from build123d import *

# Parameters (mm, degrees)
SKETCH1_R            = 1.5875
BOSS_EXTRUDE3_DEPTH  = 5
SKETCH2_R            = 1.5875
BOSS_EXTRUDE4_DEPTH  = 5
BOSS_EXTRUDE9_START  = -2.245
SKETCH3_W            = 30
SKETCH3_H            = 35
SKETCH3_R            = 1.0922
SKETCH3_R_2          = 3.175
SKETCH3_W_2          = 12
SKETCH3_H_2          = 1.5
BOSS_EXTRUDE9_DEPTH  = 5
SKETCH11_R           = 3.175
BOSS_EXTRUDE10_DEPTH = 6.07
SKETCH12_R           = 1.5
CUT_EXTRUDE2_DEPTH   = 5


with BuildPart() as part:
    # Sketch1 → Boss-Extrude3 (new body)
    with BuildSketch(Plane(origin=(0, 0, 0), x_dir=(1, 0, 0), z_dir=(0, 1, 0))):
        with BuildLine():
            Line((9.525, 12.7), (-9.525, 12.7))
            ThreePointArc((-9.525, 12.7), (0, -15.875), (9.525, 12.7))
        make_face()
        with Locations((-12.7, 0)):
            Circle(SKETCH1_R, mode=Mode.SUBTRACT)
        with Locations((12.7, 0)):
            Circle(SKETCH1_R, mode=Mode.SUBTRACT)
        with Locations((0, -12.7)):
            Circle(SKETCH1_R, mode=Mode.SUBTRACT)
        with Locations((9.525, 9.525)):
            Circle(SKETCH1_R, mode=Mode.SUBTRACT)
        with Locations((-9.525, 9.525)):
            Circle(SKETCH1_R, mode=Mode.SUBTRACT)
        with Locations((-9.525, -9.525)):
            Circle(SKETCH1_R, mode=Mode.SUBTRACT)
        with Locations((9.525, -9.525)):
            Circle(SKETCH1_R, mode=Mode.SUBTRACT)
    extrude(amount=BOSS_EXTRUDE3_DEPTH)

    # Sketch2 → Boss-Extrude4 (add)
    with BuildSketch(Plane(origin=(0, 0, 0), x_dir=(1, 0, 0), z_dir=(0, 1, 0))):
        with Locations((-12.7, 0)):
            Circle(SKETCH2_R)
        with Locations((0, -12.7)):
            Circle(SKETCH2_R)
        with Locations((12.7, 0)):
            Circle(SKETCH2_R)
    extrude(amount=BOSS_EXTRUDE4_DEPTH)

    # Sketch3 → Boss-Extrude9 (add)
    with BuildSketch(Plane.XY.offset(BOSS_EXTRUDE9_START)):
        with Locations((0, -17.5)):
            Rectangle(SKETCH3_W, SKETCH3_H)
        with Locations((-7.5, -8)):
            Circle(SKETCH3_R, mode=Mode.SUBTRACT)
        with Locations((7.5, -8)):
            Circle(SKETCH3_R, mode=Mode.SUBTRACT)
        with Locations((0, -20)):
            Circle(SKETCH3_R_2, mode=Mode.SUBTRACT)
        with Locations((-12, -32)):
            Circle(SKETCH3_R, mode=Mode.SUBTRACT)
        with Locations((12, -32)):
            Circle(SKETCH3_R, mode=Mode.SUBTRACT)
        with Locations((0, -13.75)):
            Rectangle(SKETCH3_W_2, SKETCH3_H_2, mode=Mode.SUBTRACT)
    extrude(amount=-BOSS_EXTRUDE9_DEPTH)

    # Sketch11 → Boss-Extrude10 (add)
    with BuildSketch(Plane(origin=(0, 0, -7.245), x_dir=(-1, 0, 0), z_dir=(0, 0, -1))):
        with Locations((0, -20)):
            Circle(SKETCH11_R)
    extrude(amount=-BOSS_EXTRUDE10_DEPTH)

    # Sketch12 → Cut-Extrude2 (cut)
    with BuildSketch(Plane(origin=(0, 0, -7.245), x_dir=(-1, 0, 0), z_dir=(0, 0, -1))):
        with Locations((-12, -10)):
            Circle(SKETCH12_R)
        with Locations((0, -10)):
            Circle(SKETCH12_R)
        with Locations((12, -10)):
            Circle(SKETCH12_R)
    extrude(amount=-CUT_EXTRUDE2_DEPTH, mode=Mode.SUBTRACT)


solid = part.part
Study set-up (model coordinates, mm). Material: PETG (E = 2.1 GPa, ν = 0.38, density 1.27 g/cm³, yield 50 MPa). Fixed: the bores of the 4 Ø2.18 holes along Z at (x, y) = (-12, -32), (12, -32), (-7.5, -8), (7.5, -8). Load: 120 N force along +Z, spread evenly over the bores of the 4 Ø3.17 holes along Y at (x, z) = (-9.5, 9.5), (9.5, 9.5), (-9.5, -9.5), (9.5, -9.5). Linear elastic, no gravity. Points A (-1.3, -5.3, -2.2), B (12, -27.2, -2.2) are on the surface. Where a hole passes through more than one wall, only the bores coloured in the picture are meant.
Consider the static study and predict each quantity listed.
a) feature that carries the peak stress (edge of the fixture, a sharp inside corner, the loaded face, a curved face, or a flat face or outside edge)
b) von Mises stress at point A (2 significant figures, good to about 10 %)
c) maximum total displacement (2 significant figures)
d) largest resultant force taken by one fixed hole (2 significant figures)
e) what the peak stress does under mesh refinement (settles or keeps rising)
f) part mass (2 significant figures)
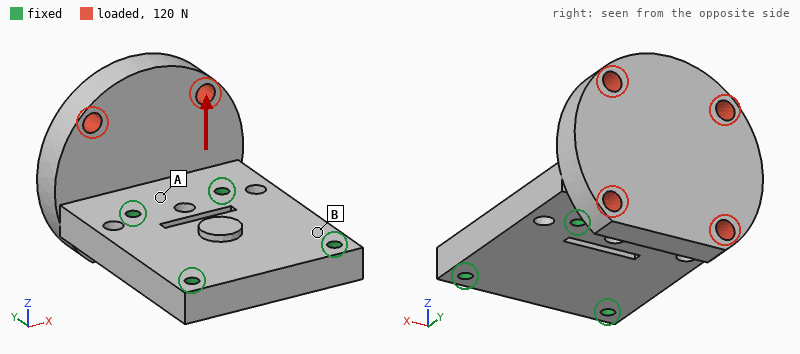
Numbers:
edge of the fixture
4.2 MPa
0.30 mm
65 N
keeps rising
11 g
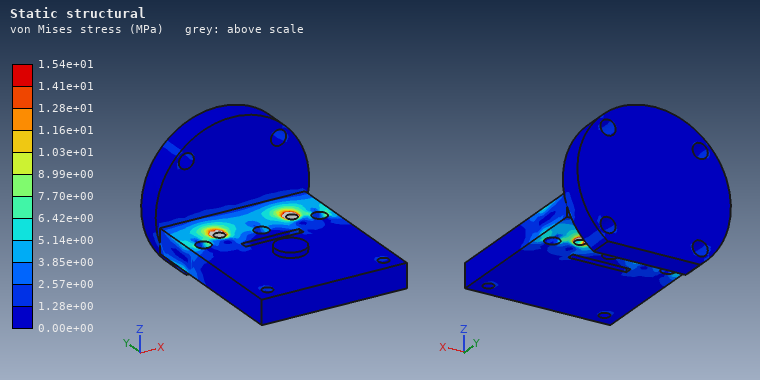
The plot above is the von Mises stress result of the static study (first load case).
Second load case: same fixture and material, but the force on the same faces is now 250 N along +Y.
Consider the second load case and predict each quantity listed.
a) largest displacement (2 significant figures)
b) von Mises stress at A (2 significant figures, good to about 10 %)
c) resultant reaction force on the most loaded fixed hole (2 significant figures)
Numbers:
0.67 mm
7.1 MPa
120 N
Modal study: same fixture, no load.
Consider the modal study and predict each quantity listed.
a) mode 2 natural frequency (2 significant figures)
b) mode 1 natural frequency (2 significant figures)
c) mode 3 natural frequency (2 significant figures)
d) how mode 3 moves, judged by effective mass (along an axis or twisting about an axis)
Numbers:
2700 Hz
1500 Hz
4100 Hz
along Z
